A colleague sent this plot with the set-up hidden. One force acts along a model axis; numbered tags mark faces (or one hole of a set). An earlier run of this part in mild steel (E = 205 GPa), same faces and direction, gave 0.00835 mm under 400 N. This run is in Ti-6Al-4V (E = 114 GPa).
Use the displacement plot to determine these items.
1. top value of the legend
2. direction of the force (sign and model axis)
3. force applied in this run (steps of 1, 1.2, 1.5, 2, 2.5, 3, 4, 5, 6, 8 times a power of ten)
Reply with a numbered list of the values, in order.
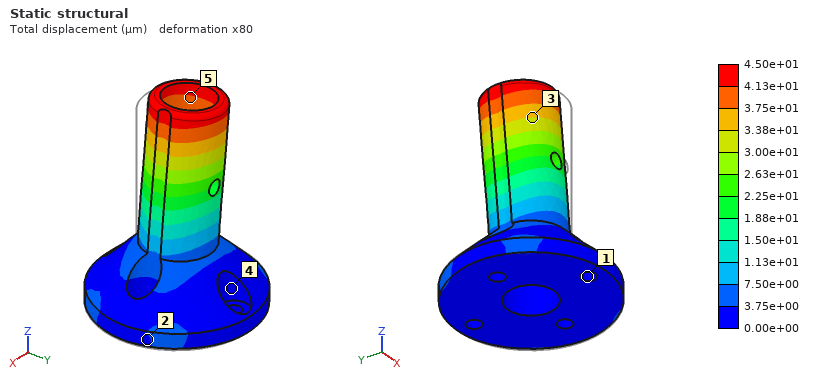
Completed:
1. 4.50e+01 µm
2. -X
3. 1.2 kN
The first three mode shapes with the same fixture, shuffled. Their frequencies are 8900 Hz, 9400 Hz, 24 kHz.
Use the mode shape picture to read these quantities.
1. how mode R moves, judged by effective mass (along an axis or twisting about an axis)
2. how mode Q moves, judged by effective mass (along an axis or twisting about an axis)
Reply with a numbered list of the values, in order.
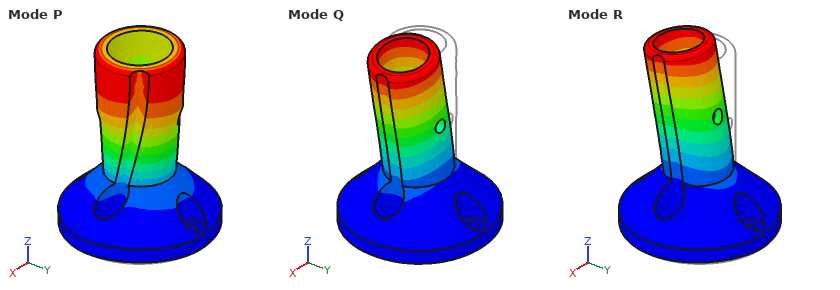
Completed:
1. along Y
2. along X
